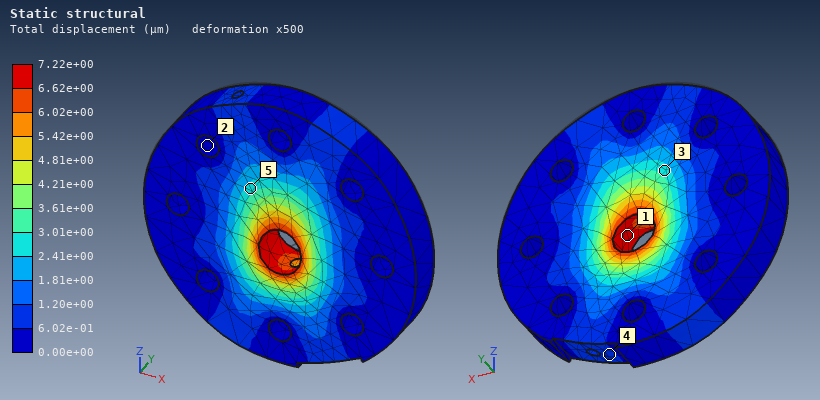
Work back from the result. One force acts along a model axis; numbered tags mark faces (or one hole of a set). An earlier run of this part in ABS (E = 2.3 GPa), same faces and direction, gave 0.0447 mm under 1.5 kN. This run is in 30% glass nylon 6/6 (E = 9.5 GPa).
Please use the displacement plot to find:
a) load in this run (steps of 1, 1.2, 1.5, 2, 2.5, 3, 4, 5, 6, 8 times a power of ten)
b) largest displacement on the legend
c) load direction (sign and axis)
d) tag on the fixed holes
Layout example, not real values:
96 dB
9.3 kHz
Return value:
1 kN
7.22e+00 µm
-Z
2
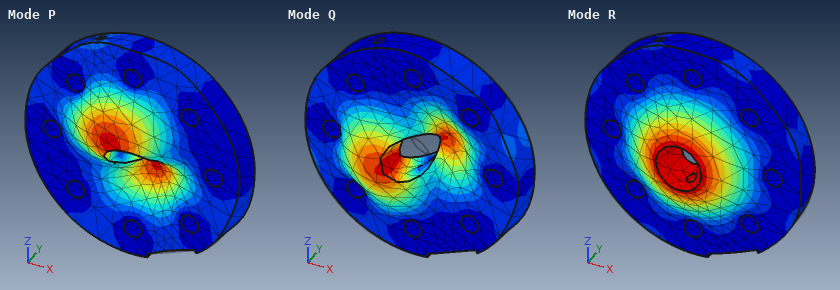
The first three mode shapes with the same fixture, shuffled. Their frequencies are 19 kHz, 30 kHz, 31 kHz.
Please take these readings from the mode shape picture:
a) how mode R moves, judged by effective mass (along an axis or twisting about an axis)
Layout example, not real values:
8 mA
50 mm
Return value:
along Y
